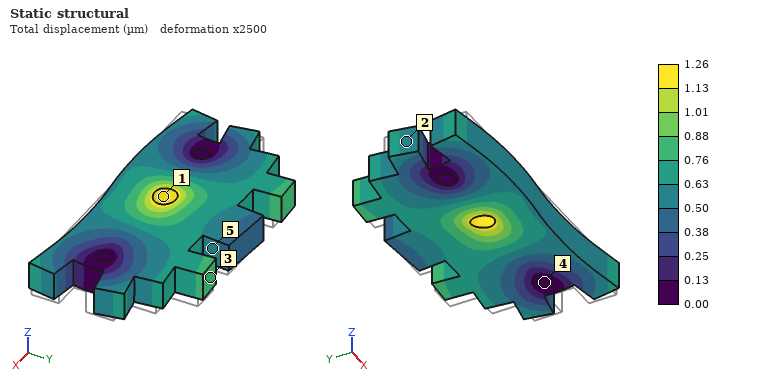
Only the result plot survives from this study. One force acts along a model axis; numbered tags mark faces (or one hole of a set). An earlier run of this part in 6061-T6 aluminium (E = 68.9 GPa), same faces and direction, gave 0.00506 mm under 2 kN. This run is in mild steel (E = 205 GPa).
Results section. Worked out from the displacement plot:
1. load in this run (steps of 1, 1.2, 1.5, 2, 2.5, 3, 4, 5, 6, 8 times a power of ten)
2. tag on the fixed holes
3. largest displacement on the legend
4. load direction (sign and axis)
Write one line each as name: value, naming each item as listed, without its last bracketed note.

load in this run: 1.5 kN
tag on the fixed holes: 4
largest displacement on the legend: 1.26 µm
load direction: -X
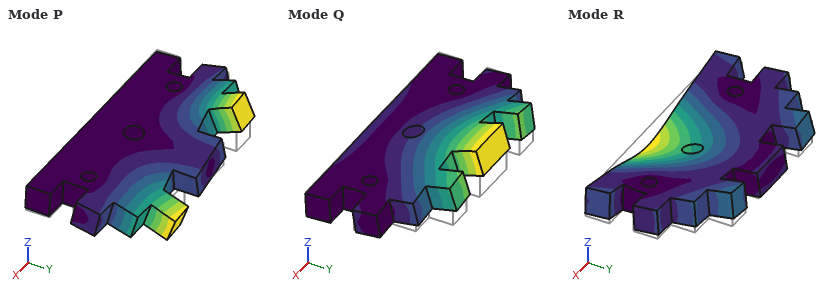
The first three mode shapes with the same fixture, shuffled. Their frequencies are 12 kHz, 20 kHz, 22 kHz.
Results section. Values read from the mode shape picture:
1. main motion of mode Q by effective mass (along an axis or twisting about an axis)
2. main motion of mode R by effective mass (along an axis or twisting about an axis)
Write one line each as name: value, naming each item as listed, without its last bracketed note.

main motion of mode Q by effective mass: along Z
main motion of mode R by effective mass: along Z
